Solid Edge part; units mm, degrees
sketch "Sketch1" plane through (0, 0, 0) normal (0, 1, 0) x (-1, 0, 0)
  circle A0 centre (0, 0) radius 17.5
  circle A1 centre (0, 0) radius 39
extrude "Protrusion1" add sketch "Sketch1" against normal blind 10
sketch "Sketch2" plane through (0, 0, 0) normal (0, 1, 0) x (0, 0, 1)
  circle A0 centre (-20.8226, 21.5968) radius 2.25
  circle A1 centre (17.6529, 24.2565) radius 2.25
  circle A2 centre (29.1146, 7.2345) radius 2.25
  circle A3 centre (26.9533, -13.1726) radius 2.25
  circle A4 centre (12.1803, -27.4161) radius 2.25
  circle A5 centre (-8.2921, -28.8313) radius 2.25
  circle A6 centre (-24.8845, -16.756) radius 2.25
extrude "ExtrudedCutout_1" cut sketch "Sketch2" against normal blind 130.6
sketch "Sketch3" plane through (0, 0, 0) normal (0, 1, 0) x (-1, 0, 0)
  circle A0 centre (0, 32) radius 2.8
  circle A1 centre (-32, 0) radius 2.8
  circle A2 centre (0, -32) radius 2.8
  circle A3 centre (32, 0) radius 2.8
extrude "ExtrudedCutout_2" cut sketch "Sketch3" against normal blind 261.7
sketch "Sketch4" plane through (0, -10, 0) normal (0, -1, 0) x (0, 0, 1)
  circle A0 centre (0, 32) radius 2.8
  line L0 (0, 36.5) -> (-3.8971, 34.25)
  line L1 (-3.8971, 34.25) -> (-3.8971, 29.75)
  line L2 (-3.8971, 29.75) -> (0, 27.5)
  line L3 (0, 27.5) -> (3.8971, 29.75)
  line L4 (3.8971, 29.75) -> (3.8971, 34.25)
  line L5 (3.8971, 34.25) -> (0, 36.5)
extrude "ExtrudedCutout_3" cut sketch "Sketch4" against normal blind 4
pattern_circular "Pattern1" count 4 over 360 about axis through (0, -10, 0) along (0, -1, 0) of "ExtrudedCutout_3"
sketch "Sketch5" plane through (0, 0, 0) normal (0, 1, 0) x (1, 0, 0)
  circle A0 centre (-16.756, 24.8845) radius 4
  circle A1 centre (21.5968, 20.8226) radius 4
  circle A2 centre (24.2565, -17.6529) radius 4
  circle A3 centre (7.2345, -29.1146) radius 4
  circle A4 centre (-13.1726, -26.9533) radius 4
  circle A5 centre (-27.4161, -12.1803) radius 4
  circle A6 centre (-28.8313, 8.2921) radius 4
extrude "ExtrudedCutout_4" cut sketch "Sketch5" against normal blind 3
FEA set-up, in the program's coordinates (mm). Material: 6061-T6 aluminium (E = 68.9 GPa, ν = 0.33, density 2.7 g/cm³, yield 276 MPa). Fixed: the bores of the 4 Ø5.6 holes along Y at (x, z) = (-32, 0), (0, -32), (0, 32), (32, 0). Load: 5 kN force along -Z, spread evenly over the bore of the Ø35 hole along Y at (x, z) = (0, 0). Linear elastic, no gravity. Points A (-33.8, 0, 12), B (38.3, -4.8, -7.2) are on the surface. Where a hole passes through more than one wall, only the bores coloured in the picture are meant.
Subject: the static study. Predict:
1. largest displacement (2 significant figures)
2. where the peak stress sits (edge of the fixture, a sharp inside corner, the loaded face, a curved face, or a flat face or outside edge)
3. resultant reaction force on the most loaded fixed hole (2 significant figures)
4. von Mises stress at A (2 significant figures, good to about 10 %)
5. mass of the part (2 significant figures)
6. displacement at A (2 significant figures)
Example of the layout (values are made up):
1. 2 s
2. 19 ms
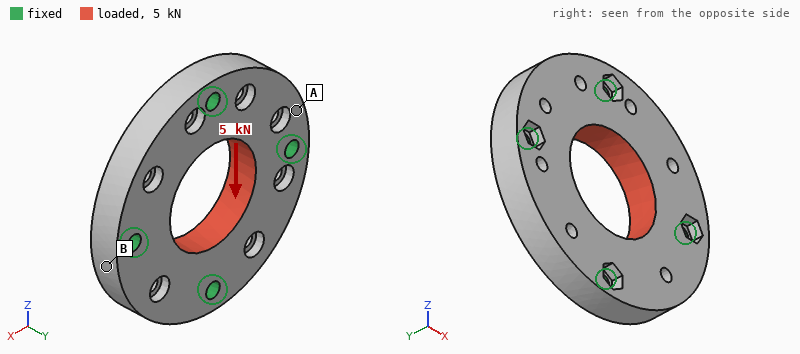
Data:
1. 3.8 µm
2. edge of the fixture
3. 1.4 kN
4. 6.1 MPa
5. 94 g
6. 1.0 µm
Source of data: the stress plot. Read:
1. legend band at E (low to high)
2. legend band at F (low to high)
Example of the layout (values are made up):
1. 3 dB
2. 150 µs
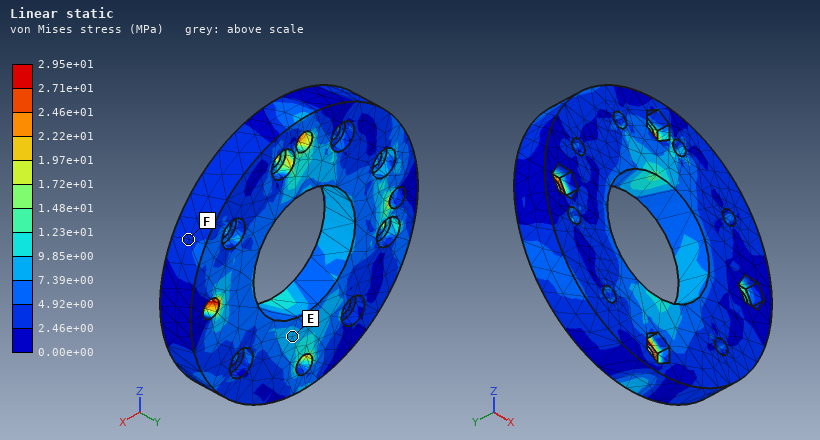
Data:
1. 7.39e+00 to 9.85e+00 MPa
2. 2.46e+00 to 4.92e+00 MPa
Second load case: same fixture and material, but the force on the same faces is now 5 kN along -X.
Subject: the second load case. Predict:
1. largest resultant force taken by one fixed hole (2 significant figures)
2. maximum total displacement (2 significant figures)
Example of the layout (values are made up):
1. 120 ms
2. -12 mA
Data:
1. 1.4 kN
2. 3.8 µm
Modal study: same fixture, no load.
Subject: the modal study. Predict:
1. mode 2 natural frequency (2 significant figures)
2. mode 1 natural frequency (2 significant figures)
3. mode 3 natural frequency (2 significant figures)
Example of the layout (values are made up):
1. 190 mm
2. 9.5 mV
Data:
1. 13 kHz
2. 12 kHz
3. 14 kHz
